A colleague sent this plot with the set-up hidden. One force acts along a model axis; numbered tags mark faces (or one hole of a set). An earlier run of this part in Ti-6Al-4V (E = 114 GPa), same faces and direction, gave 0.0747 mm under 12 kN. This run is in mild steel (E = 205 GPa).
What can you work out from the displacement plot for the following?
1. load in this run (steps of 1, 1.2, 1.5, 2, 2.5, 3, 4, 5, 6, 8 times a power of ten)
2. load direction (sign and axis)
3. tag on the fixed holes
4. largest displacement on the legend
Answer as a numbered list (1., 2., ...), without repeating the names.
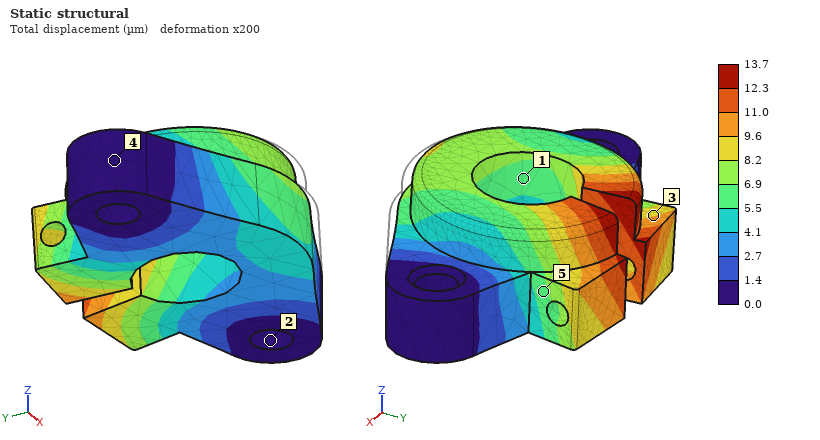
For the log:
1. 4 kN
2. +Y
3. 2
4. 13.7 µm
